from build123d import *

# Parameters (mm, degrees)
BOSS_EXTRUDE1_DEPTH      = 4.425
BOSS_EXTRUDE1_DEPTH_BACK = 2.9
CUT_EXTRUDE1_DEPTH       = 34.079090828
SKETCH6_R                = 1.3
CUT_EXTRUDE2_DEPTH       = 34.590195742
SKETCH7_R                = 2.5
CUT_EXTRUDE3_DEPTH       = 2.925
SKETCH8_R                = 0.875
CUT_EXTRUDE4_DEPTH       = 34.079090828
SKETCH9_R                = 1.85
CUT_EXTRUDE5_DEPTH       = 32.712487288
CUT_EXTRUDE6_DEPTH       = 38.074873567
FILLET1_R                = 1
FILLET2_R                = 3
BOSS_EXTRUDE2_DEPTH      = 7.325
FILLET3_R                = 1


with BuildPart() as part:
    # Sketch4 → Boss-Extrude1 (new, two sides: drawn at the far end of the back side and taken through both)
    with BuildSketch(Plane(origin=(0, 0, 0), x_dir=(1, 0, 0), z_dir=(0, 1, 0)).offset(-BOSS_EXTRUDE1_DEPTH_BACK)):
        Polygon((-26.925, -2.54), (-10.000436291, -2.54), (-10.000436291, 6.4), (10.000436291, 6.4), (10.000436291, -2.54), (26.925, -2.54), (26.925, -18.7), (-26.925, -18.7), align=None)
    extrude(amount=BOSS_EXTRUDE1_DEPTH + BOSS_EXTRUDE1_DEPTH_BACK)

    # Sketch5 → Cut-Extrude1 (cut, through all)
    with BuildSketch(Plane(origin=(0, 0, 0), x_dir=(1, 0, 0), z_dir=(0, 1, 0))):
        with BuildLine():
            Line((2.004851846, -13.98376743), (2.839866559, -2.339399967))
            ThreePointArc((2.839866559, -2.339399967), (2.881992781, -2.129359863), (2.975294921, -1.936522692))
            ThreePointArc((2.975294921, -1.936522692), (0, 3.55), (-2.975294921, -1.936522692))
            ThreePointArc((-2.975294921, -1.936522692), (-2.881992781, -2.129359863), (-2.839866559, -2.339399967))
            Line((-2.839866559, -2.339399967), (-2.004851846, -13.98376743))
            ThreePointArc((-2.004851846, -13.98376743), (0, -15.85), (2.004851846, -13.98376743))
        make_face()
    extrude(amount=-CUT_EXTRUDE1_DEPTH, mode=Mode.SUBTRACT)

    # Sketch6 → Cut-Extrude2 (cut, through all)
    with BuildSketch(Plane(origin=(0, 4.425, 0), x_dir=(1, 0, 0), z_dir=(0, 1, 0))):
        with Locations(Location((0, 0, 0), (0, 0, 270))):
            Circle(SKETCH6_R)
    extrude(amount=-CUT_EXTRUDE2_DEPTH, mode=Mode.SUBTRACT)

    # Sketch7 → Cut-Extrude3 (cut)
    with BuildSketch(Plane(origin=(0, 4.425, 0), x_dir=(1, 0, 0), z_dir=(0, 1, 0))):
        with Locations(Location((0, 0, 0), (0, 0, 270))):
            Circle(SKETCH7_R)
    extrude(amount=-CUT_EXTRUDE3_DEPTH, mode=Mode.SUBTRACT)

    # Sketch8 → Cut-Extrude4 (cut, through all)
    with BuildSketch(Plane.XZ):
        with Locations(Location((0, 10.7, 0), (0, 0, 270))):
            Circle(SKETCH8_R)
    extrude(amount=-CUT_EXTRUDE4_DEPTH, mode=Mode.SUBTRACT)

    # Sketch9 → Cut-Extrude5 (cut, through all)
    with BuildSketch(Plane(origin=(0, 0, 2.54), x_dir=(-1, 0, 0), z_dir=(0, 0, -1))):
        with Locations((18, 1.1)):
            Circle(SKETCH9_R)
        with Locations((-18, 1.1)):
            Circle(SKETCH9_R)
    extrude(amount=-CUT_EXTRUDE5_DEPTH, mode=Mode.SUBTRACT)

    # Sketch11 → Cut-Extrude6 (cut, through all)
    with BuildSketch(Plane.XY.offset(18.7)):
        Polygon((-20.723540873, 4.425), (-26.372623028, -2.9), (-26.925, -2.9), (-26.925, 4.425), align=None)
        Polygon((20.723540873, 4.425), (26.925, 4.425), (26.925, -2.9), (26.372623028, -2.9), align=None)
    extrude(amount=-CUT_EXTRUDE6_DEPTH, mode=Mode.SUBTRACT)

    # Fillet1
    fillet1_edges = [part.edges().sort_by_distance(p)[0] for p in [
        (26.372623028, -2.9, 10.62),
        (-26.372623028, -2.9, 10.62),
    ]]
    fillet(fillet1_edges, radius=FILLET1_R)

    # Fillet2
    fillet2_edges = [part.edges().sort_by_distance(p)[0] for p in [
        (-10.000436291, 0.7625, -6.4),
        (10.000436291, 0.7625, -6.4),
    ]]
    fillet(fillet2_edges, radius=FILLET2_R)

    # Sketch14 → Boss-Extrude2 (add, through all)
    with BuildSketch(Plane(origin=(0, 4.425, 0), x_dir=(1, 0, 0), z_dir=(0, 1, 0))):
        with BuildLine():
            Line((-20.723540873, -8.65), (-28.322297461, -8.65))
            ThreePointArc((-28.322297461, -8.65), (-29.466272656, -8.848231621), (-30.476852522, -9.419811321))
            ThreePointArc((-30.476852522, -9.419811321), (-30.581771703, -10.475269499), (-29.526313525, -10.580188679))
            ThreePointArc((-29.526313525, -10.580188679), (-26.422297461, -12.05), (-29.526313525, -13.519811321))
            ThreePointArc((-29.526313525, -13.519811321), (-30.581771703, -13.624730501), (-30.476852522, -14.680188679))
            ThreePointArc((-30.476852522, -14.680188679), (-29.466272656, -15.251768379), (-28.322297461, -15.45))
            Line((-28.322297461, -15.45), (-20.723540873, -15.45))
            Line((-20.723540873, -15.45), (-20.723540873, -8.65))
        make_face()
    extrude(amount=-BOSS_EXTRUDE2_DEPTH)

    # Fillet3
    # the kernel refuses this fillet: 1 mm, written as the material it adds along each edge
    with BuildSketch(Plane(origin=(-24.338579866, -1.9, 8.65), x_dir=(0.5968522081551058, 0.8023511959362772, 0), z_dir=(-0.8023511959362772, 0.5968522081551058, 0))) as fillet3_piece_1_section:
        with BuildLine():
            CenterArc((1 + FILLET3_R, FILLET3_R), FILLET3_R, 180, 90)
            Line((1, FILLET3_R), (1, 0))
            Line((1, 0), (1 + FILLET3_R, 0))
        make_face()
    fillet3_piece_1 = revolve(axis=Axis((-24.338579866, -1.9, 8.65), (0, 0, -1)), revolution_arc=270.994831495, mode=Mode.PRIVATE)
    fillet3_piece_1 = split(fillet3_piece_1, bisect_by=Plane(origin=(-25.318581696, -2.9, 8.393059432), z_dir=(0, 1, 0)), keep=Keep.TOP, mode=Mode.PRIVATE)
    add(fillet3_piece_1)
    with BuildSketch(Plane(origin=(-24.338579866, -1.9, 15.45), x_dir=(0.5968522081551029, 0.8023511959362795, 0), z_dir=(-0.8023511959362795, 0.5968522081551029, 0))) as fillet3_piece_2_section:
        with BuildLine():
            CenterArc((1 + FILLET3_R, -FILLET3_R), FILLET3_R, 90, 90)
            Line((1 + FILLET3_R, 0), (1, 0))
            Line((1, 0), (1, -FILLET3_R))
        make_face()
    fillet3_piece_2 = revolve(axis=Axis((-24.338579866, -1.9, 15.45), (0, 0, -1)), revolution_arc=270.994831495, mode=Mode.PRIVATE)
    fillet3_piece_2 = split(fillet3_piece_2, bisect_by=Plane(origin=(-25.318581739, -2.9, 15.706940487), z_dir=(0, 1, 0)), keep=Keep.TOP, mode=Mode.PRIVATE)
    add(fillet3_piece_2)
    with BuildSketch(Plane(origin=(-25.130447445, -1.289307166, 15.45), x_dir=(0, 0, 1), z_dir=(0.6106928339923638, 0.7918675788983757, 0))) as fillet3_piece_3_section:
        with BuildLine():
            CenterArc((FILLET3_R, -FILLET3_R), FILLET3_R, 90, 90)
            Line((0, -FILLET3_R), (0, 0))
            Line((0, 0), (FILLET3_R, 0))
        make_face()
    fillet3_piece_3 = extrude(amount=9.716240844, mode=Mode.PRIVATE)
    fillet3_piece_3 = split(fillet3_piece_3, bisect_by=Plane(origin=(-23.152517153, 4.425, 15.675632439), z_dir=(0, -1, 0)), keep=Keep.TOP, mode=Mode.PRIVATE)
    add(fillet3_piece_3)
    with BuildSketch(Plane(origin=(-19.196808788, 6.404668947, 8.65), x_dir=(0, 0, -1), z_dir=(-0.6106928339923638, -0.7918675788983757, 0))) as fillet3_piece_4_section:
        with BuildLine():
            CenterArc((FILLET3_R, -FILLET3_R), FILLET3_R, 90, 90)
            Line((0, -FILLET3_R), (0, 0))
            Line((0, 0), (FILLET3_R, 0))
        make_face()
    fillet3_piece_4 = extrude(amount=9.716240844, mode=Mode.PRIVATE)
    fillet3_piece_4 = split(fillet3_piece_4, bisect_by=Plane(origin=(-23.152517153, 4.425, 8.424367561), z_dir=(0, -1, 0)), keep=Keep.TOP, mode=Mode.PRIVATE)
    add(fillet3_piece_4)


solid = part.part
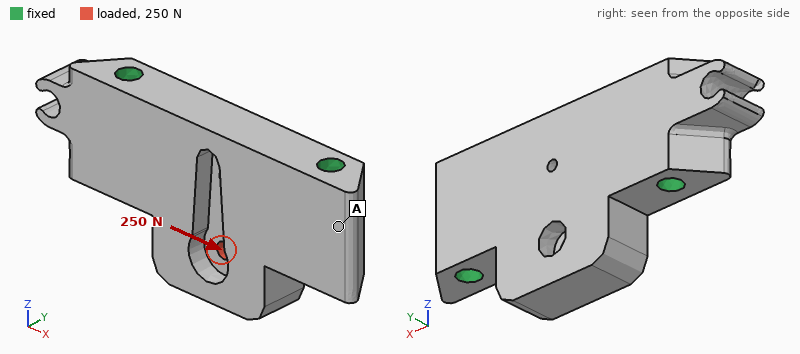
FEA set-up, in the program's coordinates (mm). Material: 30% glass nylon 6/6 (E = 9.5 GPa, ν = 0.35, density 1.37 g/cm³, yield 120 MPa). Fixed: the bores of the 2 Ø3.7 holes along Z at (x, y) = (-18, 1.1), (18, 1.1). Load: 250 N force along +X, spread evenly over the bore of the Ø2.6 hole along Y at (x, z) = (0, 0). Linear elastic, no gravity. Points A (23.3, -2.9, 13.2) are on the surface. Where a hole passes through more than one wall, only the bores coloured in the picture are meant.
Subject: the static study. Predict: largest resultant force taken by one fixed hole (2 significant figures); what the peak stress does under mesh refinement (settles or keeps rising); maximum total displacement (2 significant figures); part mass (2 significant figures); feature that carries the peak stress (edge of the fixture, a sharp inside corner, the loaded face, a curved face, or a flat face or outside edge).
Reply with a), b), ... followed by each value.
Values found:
a) 140 N
b) keeps rising
c) 12 µm
d) 8.7 g
e) a sharp inside corner
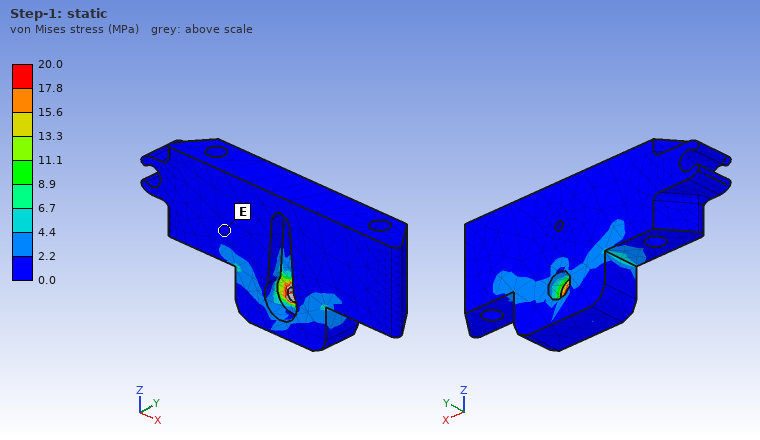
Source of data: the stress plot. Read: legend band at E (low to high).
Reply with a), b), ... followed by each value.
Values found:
a) 0.0 to 2.2 MPa
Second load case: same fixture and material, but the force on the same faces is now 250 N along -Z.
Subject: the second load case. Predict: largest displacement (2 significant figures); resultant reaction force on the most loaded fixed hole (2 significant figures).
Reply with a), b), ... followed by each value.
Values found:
a) 12 µm
b) 130 N
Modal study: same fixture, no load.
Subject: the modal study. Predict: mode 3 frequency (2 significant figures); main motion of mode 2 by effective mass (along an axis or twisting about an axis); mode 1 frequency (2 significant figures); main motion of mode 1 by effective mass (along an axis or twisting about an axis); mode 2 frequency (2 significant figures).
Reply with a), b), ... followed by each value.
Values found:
a) 17 kHz
b) along Y
c) 7600 Hz
d) along Y
e) 13 kHz
